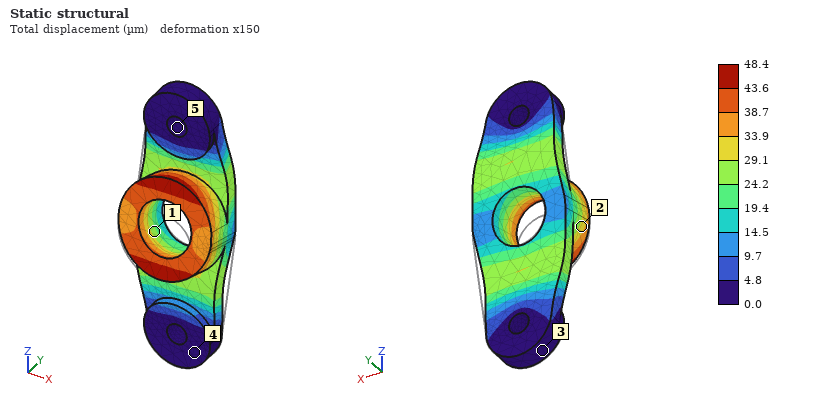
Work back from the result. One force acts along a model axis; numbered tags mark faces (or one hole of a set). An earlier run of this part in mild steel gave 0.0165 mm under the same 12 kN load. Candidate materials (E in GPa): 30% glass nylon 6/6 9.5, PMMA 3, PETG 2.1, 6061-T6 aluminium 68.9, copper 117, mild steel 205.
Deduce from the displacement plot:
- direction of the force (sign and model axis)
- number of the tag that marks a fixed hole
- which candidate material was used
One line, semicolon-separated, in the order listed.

+Z; 5; 6061-T6 aluminium
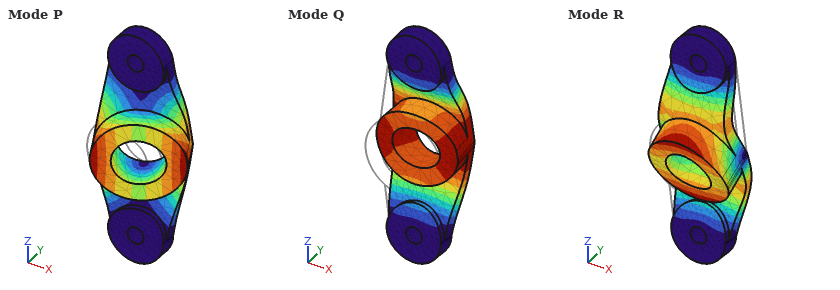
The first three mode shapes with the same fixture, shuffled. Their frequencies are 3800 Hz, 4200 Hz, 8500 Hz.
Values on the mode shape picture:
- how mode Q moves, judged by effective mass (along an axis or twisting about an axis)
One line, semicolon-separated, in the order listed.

along Y
